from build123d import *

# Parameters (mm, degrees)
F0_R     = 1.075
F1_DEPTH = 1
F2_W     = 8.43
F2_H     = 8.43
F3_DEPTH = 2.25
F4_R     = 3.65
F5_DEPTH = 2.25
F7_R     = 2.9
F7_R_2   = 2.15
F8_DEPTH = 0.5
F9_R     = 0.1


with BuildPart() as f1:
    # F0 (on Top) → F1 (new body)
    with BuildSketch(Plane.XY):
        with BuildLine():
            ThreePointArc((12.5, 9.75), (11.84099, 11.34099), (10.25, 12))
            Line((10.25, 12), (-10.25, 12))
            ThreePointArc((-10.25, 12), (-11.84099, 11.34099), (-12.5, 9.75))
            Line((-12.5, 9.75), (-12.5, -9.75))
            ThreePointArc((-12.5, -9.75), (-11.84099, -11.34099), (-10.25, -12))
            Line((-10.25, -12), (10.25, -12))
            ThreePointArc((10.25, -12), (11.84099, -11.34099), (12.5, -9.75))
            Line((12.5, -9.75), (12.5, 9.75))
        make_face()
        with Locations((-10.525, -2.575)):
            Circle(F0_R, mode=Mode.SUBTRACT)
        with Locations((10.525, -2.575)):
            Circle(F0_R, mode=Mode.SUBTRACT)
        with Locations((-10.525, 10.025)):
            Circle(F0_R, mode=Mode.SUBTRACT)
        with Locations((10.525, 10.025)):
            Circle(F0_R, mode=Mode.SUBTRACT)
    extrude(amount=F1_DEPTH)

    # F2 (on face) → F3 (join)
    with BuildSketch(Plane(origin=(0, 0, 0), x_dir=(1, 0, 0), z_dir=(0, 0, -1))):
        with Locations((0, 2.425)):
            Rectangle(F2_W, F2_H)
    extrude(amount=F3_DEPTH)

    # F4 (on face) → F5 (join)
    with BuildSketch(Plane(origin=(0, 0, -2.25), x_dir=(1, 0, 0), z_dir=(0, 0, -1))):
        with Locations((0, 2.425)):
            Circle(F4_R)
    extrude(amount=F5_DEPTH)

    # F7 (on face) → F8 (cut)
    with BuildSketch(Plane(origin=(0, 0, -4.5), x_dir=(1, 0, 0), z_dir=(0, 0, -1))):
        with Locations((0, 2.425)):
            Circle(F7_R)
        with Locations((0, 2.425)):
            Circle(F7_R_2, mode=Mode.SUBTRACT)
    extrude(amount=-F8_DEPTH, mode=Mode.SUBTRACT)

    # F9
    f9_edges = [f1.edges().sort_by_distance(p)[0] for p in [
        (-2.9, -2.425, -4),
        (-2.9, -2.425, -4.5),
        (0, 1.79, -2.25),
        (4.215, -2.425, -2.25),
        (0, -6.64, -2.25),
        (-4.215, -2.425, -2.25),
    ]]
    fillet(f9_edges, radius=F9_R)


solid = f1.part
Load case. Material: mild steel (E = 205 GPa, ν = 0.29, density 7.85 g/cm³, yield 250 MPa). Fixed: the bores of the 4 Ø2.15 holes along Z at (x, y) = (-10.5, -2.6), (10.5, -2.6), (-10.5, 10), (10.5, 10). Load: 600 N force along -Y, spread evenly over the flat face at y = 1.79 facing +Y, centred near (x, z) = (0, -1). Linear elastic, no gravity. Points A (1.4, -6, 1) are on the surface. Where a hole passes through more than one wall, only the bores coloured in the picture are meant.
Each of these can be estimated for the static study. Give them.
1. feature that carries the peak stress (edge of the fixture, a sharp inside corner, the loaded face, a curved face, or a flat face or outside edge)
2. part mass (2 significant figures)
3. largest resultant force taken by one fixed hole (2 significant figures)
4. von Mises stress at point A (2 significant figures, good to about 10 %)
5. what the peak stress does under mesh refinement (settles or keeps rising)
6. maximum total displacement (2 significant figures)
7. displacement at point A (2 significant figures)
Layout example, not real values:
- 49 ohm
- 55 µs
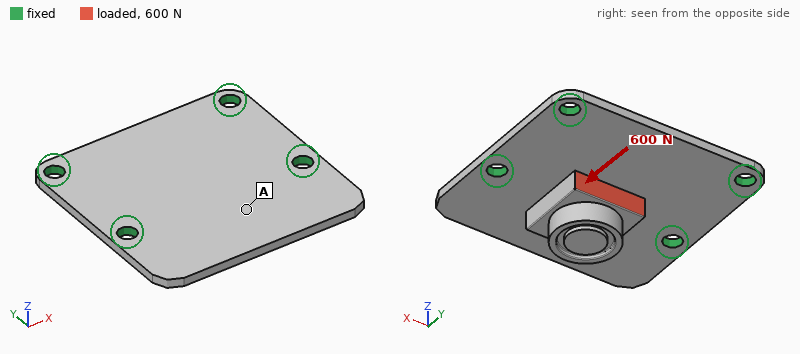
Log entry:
- edge of the fixture
- 6.5 g
- 190 N
- 21 MPa
- keeps rising
- 33 µm
- 14 µm
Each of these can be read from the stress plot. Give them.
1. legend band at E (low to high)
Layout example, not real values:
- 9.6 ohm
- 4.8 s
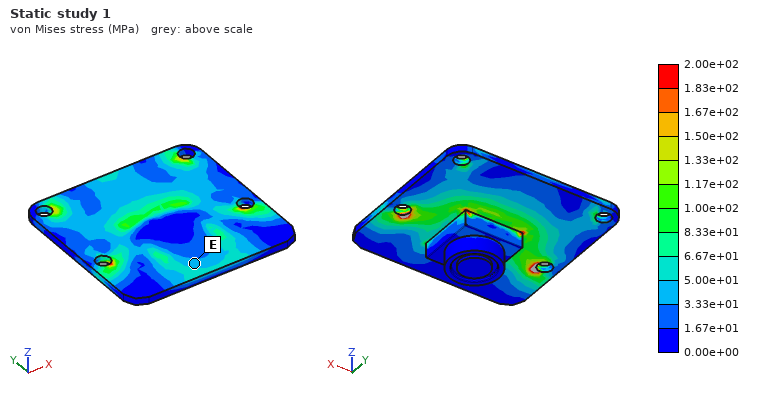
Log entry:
- 3.33e+01 to 5.00e+01 MPa
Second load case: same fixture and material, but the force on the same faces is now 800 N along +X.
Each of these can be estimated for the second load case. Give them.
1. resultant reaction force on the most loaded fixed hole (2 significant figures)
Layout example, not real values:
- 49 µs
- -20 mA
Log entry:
- 300 N
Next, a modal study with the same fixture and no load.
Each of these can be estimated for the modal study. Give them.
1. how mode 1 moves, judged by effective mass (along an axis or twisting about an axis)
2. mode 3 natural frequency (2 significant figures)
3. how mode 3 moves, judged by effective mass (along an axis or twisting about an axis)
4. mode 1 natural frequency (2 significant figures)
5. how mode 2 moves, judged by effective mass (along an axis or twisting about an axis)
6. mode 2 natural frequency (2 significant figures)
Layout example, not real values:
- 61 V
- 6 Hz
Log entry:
- along Z
- 16 kHz
- twisting about Y
- 8100 Hz
- along Z
- 11 kHz
